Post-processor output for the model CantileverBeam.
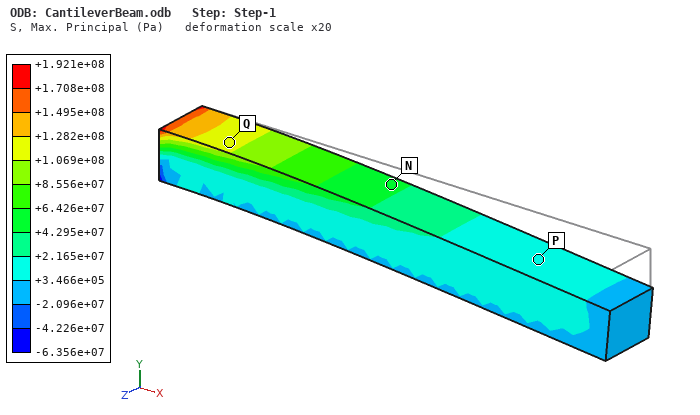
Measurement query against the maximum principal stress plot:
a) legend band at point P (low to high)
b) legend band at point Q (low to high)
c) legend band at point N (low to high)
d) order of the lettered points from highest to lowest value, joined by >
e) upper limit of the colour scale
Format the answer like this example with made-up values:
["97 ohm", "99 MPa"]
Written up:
["+3.466e+05 to +2.165e+07 Pa", "+1.069e+08 to +1.282e+08 Pa", "+4.295e+07 to +6.426e+07 Pa", "Q > N > P", "+1.921e+08 Pa"]
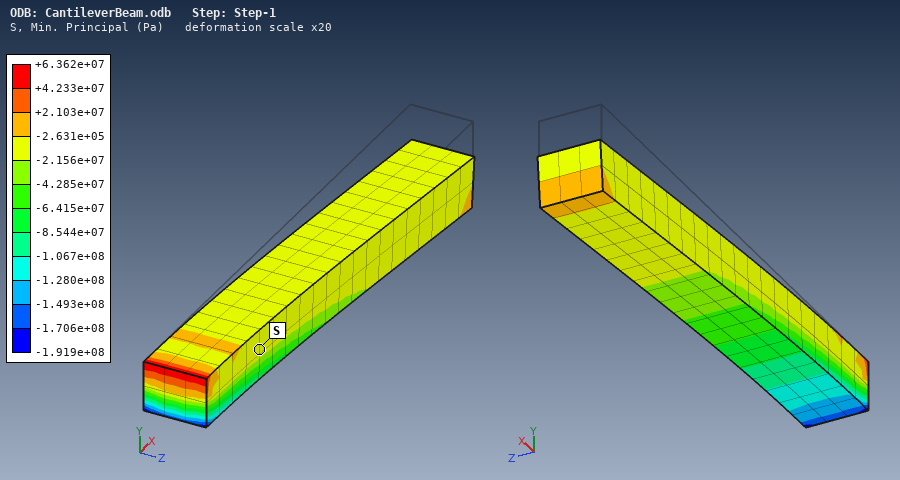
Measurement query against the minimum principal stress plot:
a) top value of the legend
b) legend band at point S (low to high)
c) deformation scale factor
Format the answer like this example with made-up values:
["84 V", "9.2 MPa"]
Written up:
["+6.362e+07 Pa", "-2.156e+07 to -2.631e+05 Pa", "20"]
